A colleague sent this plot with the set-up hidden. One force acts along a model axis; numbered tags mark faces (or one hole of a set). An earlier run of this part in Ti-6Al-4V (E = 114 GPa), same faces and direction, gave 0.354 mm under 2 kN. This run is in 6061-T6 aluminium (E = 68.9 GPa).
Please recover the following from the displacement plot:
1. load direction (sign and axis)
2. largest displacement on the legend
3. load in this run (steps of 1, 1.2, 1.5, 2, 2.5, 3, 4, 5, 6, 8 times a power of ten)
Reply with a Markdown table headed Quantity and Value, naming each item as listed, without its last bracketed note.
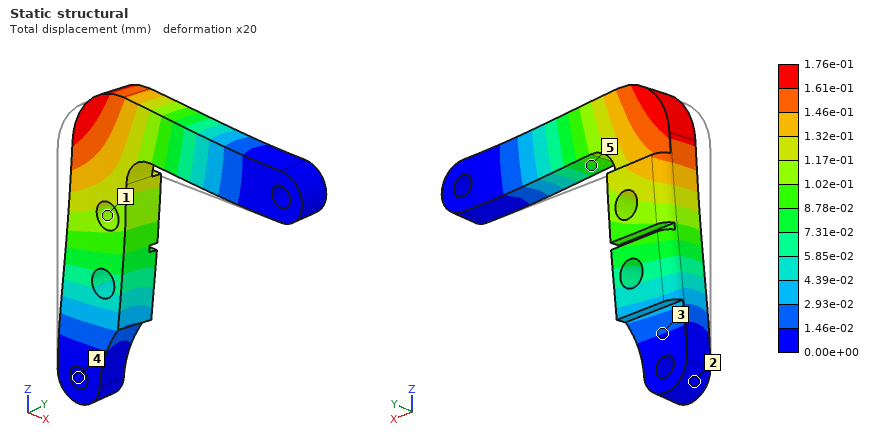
| Quantity | Value |
|---|---|
| load direction | +Y |
| largest displacement on the legend | 1.76e-01 mm |
| load in this run | 600 N |
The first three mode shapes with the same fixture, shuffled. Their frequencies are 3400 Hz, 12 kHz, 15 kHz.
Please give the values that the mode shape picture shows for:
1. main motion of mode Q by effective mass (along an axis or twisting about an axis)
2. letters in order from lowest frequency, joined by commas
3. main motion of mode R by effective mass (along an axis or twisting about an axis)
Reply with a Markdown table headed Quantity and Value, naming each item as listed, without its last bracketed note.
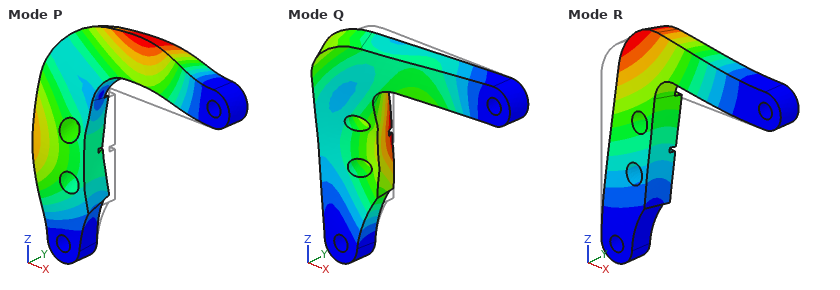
| Quantity | Value |
|---|---|
| main motion of mode Q by effective mass | along X |
| letters in order from lowest frequency, joined by commas | R, P, Q |
| main motion of mode R by effective mass | along Y |
